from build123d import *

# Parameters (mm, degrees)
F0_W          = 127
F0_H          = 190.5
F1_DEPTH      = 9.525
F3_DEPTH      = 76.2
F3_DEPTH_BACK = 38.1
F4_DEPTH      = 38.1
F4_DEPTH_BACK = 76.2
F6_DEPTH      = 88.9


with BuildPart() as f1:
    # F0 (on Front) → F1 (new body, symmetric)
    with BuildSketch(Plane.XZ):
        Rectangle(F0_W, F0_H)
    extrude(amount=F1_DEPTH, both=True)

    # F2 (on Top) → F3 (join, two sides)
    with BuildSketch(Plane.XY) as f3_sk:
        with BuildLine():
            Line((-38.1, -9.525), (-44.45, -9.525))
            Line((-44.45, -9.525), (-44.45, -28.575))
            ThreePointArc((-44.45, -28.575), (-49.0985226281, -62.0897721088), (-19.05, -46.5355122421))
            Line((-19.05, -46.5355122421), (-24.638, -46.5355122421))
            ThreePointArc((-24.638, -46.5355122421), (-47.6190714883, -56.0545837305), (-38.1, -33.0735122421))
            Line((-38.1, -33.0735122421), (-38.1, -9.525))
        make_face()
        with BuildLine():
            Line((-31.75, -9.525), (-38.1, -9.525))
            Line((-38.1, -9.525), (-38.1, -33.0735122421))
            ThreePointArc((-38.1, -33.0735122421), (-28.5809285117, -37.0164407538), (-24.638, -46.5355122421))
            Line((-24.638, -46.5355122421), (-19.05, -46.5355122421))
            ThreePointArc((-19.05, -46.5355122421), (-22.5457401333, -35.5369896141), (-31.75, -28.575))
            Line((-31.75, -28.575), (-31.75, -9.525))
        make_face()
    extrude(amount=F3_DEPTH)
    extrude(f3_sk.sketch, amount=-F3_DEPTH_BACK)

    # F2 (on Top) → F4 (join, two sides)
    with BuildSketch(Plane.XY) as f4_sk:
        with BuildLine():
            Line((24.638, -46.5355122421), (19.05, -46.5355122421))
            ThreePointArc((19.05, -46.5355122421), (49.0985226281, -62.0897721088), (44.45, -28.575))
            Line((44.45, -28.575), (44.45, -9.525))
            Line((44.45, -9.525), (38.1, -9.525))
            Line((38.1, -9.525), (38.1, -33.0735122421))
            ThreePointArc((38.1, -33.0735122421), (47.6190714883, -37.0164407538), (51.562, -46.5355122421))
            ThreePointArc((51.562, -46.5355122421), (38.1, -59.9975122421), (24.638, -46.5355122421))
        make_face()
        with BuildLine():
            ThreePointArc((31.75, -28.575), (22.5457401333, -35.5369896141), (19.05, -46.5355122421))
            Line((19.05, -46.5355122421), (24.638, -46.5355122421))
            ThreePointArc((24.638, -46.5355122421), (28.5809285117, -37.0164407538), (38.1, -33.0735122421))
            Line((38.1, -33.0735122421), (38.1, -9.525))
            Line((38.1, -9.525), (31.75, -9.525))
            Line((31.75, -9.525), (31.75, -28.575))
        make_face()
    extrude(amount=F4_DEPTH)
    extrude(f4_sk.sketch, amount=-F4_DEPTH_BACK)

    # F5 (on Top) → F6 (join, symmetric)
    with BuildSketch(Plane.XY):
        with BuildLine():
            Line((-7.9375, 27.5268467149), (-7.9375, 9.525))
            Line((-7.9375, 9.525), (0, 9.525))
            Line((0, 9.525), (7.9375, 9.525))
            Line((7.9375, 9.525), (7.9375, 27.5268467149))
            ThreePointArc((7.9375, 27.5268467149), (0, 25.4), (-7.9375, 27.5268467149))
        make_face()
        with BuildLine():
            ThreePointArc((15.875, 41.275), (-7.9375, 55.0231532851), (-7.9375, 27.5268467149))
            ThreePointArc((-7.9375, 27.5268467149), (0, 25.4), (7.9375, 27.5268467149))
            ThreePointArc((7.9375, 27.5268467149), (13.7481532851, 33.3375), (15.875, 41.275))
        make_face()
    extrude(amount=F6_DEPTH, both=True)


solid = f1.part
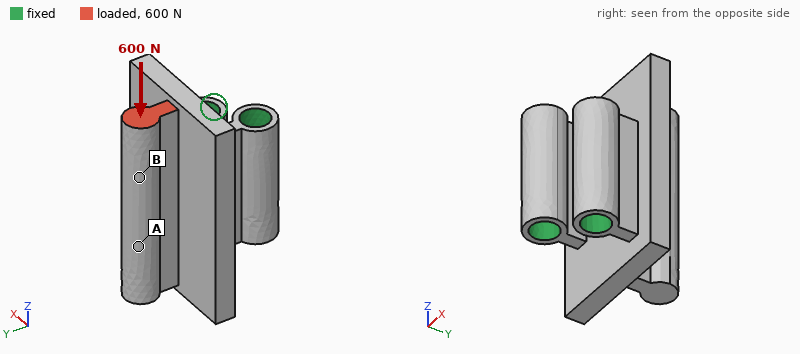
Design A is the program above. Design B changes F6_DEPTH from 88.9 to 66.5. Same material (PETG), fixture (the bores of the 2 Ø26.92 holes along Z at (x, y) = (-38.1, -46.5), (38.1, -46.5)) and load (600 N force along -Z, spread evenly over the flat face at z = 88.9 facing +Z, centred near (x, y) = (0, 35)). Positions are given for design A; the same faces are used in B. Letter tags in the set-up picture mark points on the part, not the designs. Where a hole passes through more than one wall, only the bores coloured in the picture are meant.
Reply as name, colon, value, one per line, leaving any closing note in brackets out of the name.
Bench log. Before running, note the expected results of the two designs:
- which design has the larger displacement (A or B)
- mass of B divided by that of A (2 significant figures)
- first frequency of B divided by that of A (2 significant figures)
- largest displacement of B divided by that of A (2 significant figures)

which design has the larger displacement: A
mass of B divided by that of A: 0.94
first frequency of B divided by that of A: 1.1
largest displacement of B divided by that of A: 0.86
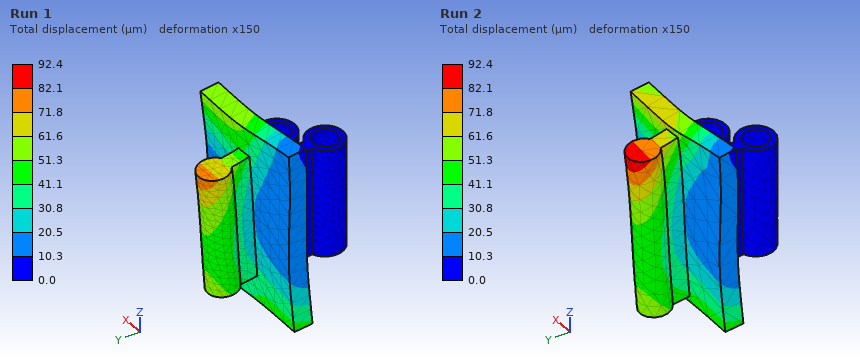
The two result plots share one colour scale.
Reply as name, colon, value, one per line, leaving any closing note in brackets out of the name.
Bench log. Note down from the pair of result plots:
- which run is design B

which run is design B: Run 1
